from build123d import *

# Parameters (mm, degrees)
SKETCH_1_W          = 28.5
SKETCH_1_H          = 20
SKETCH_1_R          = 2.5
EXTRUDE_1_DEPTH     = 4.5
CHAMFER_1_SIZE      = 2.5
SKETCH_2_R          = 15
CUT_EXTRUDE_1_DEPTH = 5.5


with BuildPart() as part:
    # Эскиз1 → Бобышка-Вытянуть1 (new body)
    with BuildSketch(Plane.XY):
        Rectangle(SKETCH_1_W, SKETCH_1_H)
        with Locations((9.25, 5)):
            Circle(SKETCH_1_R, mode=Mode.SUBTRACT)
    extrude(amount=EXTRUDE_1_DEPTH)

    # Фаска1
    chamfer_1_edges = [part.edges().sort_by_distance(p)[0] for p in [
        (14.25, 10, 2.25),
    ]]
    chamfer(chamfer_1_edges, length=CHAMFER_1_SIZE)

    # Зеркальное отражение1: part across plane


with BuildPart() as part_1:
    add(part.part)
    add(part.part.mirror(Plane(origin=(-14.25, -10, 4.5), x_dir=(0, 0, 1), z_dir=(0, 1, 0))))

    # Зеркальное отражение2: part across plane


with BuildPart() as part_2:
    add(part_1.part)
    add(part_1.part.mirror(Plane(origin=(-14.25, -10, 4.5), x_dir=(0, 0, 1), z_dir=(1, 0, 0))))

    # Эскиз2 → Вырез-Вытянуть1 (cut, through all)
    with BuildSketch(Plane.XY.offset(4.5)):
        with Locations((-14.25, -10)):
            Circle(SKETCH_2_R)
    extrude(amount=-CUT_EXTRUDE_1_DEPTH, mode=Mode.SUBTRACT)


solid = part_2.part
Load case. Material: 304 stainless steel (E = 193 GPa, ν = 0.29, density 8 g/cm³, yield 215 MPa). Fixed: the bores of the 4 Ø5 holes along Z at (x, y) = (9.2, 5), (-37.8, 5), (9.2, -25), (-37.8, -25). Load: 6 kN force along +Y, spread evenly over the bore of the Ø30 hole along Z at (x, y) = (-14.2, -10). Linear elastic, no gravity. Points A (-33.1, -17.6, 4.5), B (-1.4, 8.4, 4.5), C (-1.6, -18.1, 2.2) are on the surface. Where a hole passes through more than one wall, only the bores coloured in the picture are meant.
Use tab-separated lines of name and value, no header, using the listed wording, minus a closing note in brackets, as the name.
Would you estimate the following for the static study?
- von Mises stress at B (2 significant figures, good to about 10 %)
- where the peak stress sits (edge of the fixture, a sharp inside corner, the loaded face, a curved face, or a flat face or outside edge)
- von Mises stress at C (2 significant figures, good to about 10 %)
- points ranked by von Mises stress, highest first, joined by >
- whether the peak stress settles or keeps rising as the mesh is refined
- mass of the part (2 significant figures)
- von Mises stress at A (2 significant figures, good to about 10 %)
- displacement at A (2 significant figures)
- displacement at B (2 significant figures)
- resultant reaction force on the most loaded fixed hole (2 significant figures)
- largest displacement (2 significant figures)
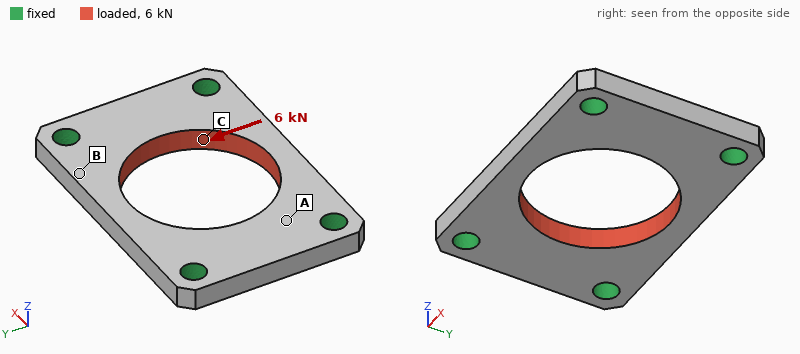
von Mises stress at B	12 MPa
where the peak stress sits	edge of the fixture
von Mises stress at C	73 MPa
points ranked by von Mises stress, highest first, joined by >	C > A > B
whether the peak stress settles or keeps rising as the mesh is refined	keeps rising
mass of the part	53 g
von Mises stress at A	39 MPa
displacement at A	1.8 µm
displacement at B	4.2 µm
resultant reaction force on the most loaded fixed hole	1.6 kN
largest displacement	11 µm
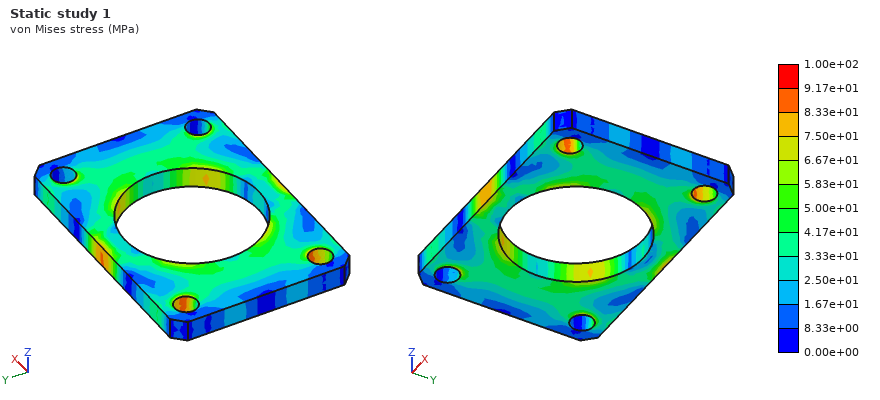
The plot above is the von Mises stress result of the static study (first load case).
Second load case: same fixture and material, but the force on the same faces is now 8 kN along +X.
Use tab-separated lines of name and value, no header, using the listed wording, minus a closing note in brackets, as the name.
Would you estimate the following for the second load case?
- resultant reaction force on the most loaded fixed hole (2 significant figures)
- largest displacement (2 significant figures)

resultant reaction force on the most loaded fixed hole	2.0 kN
largest displacement	3.4 µm
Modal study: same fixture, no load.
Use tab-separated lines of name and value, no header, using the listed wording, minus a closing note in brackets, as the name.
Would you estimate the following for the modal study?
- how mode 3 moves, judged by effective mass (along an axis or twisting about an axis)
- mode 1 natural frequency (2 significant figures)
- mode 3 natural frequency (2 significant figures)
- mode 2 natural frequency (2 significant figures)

how mode 3 moves, judged by effective mass	twisting about Y
mode 1 natural frequency	13 kHz
mode 3 natural frequency	23 kHz
mode 2 natural frequency	13 kHz
